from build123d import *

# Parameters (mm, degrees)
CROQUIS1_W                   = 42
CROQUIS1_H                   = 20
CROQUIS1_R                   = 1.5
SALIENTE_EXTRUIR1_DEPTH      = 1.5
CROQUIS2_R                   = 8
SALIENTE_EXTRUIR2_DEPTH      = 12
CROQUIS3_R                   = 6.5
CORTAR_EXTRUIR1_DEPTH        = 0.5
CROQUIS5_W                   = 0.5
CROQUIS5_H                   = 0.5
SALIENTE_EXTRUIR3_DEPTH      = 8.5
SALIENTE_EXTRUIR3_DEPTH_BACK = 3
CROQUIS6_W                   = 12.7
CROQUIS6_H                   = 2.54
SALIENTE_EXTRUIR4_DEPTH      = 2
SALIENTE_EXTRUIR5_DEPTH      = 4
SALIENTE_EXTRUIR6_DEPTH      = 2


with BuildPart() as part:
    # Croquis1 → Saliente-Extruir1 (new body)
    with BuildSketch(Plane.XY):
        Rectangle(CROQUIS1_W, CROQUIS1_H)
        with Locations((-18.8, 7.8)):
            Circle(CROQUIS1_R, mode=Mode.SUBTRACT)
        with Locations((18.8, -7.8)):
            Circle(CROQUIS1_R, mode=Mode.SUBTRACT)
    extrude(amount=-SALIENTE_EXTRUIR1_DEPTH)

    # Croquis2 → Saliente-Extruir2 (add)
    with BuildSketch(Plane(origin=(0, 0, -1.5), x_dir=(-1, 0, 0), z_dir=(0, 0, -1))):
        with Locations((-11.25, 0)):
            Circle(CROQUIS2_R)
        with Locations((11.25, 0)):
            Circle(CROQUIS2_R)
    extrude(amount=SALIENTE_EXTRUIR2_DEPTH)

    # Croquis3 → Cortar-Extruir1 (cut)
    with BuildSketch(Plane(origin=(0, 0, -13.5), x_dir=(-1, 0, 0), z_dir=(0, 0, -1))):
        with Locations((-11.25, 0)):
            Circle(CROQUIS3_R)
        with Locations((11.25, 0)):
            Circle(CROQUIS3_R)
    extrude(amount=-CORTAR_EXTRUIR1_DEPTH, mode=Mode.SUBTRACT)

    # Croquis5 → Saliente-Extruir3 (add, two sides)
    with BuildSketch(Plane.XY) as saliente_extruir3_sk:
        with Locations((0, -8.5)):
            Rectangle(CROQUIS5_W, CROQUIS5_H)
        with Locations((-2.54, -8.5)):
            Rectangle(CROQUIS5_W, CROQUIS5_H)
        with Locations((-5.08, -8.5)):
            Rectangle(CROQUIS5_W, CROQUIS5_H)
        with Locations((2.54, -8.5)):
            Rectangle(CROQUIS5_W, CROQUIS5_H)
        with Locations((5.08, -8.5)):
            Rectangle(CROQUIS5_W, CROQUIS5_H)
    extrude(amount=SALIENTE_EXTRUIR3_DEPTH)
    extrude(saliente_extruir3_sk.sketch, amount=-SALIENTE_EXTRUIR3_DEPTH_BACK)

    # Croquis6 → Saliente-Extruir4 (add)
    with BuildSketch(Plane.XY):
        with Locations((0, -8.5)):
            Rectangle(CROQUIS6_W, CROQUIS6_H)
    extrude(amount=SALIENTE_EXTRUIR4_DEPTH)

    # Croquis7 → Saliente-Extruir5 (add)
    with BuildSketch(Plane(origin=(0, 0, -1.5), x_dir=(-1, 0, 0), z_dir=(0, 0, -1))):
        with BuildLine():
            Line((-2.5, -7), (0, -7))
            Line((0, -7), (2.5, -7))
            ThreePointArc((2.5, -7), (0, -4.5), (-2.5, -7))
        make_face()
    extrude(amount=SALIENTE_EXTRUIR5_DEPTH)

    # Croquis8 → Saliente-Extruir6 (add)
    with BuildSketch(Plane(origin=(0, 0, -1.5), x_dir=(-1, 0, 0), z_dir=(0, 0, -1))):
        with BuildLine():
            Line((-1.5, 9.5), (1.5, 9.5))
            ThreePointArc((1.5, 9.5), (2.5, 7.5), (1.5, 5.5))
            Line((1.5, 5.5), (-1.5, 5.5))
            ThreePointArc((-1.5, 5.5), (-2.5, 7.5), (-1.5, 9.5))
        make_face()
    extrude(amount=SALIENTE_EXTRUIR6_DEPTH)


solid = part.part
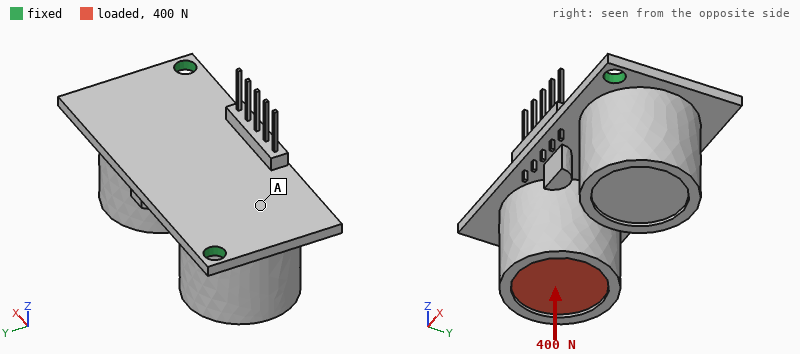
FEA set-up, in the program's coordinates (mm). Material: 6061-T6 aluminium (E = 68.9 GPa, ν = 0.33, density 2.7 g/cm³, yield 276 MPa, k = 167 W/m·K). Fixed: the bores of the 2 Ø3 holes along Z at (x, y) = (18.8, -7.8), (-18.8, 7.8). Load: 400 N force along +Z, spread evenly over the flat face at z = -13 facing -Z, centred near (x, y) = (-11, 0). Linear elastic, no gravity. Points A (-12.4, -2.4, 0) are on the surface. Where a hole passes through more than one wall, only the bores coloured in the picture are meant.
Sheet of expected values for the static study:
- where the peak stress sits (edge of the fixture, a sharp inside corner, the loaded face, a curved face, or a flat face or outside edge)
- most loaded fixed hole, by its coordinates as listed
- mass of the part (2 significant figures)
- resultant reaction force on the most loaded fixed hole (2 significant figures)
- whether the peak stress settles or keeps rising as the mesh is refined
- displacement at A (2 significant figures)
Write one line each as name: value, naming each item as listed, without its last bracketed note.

where the peak stress sits: edge of the fixture
most loaded fixed hole, by its coordinates as listed: (-18.8, 7.8)
mass of the part: 16 g
resultant reaction force on the most loaded fixed hole: 310 N
whether the peak stress settles or keeps rising as the mesh is refined: keeps rising
displacement at A: 0.11 mm
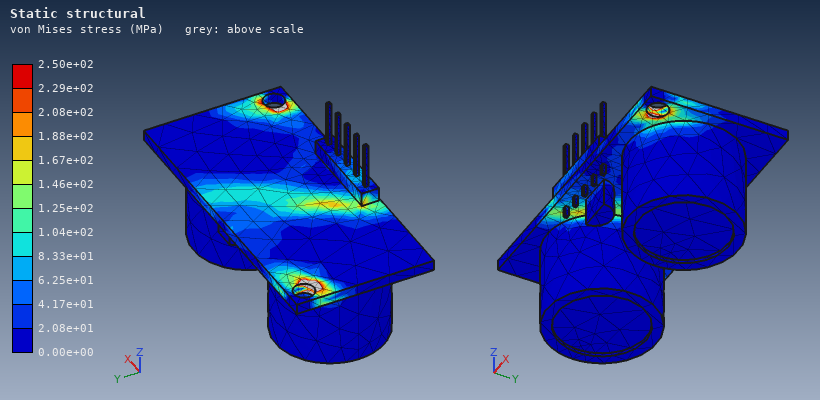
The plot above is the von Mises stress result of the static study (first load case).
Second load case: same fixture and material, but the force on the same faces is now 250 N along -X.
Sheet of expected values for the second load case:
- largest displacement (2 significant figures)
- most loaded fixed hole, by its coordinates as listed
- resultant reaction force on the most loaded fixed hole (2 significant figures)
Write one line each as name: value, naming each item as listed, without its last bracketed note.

largest displacement: 0.15 mm
most loaded fixed hole, by its coordinates as listed: (-18.8, 7.8)
resultant reaction force on the most loaded fixed hole: 180 N
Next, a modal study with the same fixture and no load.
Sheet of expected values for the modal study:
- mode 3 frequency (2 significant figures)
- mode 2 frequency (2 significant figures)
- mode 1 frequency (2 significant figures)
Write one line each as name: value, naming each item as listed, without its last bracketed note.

mode 3 frequency: 4200 Hz
mode 2 frequency: 2300 Hz
mode 1 frequency: 2200 Hz
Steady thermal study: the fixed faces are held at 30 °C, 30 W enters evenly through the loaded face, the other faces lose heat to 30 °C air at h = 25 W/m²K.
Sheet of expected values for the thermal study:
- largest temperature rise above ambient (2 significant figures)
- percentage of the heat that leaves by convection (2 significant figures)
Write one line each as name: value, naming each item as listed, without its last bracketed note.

largest temperature rise above ambient: 49 K
percentage of the heat that leaves by convection: 7.2 %
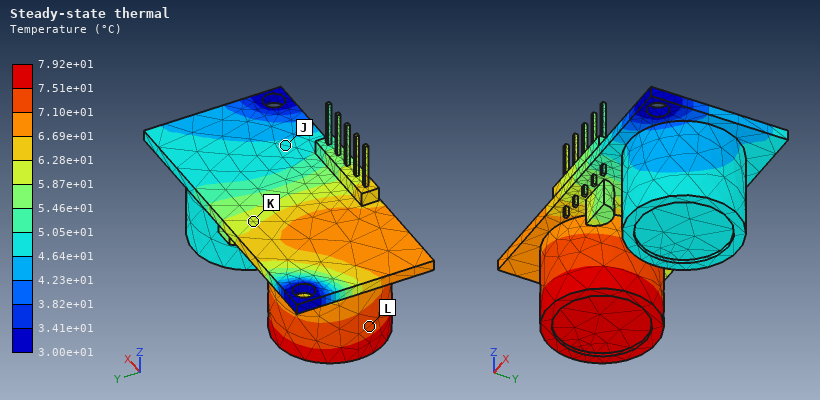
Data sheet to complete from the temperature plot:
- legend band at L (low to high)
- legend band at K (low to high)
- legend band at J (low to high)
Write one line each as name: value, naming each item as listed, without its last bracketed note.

legend band at L: 7.10e+01 to 7.51e+01 °C
legend band at K: 5.87e+01 to 6.28e+01 °C
legend band at J: 4.64e+01 to 5.05e+01 °C
